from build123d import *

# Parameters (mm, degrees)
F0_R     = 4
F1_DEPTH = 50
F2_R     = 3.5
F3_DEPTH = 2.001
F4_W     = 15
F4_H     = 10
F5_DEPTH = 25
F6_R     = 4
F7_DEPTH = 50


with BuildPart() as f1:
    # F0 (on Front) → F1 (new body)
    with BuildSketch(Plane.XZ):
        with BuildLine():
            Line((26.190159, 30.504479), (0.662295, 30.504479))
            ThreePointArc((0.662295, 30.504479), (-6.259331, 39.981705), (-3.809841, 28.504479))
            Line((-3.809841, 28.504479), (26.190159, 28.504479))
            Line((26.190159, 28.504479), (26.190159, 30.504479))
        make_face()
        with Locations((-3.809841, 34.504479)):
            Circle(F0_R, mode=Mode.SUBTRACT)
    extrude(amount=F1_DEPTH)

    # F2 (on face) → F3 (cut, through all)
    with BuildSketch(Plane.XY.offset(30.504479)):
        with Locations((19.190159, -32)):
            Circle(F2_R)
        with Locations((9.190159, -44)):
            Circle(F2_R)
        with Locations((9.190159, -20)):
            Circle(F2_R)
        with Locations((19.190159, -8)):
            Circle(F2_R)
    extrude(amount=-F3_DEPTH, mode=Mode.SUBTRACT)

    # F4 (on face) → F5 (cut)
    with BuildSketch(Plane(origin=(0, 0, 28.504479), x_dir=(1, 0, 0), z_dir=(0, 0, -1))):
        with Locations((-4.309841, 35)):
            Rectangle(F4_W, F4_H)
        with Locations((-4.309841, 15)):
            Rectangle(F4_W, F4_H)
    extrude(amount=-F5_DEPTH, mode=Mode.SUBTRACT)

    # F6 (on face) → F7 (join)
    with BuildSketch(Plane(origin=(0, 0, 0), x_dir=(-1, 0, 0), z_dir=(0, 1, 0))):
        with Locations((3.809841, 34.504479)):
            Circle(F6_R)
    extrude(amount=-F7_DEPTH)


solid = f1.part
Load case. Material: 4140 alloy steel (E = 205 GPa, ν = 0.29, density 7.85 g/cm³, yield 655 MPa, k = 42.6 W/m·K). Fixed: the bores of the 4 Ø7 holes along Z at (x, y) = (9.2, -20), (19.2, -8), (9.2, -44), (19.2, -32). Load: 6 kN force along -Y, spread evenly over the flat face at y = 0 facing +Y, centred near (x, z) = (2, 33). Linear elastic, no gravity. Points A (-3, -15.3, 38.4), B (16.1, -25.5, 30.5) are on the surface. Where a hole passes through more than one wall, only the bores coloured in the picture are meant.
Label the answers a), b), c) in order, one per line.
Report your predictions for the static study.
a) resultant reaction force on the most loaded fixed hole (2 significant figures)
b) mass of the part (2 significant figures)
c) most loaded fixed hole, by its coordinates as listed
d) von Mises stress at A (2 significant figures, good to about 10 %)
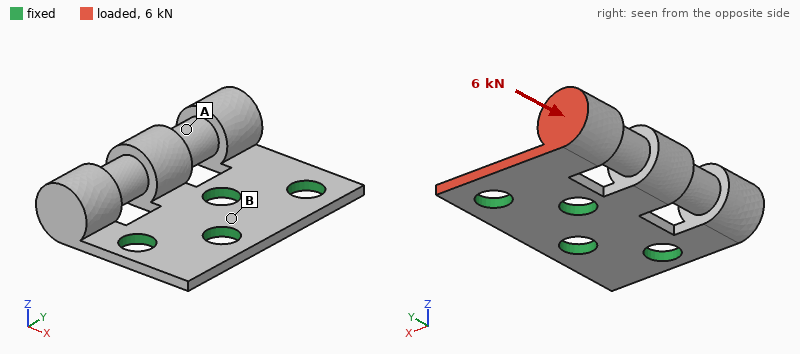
a) 3.2 kN
b) 52 g
c) (9.2, -20)
d) 89 MPa
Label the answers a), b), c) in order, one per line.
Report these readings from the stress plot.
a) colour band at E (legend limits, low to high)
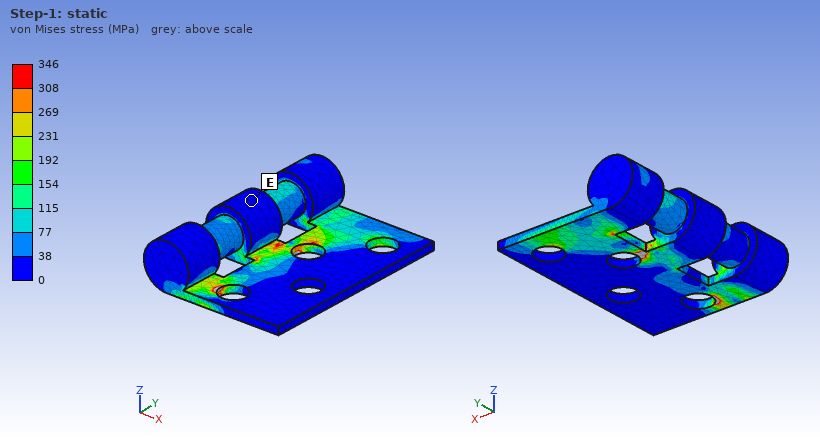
a) 0 to 38 MPa
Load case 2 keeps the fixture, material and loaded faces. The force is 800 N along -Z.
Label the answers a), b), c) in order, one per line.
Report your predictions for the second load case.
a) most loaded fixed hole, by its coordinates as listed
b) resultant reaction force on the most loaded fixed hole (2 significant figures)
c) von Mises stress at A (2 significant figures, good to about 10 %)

a) (9.2, -20)
b) 1.1 kN
c) 100 MPa
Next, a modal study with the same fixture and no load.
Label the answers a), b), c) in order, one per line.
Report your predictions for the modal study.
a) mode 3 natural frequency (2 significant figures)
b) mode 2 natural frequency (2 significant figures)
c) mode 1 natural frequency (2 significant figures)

a) 11 kHz
b) 5100 Hz
c) 2100 Hz
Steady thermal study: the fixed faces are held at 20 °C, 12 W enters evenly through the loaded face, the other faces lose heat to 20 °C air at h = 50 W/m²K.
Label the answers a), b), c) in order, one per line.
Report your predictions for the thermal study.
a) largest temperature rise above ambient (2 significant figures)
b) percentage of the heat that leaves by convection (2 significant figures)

a) 60 K
b) 26 %
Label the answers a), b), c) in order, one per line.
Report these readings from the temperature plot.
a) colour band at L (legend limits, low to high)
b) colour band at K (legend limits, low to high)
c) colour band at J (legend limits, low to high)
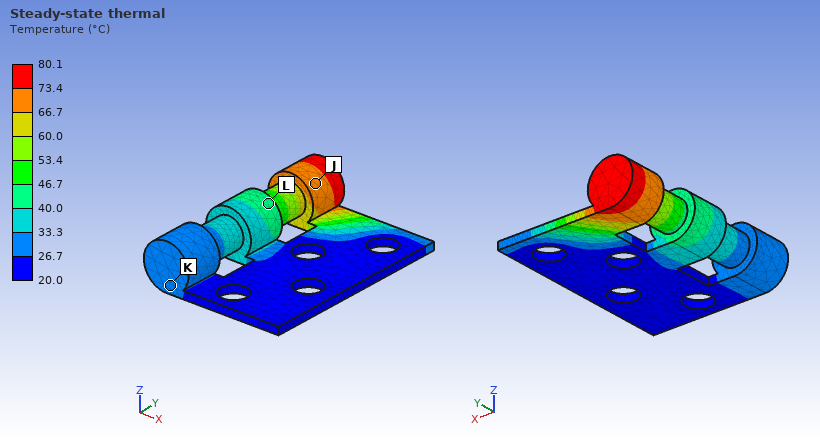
a) 40.0 to 46.7 °C
b) 26.7 to 33.3 °C
c) 66.7 to 73.4 °C
